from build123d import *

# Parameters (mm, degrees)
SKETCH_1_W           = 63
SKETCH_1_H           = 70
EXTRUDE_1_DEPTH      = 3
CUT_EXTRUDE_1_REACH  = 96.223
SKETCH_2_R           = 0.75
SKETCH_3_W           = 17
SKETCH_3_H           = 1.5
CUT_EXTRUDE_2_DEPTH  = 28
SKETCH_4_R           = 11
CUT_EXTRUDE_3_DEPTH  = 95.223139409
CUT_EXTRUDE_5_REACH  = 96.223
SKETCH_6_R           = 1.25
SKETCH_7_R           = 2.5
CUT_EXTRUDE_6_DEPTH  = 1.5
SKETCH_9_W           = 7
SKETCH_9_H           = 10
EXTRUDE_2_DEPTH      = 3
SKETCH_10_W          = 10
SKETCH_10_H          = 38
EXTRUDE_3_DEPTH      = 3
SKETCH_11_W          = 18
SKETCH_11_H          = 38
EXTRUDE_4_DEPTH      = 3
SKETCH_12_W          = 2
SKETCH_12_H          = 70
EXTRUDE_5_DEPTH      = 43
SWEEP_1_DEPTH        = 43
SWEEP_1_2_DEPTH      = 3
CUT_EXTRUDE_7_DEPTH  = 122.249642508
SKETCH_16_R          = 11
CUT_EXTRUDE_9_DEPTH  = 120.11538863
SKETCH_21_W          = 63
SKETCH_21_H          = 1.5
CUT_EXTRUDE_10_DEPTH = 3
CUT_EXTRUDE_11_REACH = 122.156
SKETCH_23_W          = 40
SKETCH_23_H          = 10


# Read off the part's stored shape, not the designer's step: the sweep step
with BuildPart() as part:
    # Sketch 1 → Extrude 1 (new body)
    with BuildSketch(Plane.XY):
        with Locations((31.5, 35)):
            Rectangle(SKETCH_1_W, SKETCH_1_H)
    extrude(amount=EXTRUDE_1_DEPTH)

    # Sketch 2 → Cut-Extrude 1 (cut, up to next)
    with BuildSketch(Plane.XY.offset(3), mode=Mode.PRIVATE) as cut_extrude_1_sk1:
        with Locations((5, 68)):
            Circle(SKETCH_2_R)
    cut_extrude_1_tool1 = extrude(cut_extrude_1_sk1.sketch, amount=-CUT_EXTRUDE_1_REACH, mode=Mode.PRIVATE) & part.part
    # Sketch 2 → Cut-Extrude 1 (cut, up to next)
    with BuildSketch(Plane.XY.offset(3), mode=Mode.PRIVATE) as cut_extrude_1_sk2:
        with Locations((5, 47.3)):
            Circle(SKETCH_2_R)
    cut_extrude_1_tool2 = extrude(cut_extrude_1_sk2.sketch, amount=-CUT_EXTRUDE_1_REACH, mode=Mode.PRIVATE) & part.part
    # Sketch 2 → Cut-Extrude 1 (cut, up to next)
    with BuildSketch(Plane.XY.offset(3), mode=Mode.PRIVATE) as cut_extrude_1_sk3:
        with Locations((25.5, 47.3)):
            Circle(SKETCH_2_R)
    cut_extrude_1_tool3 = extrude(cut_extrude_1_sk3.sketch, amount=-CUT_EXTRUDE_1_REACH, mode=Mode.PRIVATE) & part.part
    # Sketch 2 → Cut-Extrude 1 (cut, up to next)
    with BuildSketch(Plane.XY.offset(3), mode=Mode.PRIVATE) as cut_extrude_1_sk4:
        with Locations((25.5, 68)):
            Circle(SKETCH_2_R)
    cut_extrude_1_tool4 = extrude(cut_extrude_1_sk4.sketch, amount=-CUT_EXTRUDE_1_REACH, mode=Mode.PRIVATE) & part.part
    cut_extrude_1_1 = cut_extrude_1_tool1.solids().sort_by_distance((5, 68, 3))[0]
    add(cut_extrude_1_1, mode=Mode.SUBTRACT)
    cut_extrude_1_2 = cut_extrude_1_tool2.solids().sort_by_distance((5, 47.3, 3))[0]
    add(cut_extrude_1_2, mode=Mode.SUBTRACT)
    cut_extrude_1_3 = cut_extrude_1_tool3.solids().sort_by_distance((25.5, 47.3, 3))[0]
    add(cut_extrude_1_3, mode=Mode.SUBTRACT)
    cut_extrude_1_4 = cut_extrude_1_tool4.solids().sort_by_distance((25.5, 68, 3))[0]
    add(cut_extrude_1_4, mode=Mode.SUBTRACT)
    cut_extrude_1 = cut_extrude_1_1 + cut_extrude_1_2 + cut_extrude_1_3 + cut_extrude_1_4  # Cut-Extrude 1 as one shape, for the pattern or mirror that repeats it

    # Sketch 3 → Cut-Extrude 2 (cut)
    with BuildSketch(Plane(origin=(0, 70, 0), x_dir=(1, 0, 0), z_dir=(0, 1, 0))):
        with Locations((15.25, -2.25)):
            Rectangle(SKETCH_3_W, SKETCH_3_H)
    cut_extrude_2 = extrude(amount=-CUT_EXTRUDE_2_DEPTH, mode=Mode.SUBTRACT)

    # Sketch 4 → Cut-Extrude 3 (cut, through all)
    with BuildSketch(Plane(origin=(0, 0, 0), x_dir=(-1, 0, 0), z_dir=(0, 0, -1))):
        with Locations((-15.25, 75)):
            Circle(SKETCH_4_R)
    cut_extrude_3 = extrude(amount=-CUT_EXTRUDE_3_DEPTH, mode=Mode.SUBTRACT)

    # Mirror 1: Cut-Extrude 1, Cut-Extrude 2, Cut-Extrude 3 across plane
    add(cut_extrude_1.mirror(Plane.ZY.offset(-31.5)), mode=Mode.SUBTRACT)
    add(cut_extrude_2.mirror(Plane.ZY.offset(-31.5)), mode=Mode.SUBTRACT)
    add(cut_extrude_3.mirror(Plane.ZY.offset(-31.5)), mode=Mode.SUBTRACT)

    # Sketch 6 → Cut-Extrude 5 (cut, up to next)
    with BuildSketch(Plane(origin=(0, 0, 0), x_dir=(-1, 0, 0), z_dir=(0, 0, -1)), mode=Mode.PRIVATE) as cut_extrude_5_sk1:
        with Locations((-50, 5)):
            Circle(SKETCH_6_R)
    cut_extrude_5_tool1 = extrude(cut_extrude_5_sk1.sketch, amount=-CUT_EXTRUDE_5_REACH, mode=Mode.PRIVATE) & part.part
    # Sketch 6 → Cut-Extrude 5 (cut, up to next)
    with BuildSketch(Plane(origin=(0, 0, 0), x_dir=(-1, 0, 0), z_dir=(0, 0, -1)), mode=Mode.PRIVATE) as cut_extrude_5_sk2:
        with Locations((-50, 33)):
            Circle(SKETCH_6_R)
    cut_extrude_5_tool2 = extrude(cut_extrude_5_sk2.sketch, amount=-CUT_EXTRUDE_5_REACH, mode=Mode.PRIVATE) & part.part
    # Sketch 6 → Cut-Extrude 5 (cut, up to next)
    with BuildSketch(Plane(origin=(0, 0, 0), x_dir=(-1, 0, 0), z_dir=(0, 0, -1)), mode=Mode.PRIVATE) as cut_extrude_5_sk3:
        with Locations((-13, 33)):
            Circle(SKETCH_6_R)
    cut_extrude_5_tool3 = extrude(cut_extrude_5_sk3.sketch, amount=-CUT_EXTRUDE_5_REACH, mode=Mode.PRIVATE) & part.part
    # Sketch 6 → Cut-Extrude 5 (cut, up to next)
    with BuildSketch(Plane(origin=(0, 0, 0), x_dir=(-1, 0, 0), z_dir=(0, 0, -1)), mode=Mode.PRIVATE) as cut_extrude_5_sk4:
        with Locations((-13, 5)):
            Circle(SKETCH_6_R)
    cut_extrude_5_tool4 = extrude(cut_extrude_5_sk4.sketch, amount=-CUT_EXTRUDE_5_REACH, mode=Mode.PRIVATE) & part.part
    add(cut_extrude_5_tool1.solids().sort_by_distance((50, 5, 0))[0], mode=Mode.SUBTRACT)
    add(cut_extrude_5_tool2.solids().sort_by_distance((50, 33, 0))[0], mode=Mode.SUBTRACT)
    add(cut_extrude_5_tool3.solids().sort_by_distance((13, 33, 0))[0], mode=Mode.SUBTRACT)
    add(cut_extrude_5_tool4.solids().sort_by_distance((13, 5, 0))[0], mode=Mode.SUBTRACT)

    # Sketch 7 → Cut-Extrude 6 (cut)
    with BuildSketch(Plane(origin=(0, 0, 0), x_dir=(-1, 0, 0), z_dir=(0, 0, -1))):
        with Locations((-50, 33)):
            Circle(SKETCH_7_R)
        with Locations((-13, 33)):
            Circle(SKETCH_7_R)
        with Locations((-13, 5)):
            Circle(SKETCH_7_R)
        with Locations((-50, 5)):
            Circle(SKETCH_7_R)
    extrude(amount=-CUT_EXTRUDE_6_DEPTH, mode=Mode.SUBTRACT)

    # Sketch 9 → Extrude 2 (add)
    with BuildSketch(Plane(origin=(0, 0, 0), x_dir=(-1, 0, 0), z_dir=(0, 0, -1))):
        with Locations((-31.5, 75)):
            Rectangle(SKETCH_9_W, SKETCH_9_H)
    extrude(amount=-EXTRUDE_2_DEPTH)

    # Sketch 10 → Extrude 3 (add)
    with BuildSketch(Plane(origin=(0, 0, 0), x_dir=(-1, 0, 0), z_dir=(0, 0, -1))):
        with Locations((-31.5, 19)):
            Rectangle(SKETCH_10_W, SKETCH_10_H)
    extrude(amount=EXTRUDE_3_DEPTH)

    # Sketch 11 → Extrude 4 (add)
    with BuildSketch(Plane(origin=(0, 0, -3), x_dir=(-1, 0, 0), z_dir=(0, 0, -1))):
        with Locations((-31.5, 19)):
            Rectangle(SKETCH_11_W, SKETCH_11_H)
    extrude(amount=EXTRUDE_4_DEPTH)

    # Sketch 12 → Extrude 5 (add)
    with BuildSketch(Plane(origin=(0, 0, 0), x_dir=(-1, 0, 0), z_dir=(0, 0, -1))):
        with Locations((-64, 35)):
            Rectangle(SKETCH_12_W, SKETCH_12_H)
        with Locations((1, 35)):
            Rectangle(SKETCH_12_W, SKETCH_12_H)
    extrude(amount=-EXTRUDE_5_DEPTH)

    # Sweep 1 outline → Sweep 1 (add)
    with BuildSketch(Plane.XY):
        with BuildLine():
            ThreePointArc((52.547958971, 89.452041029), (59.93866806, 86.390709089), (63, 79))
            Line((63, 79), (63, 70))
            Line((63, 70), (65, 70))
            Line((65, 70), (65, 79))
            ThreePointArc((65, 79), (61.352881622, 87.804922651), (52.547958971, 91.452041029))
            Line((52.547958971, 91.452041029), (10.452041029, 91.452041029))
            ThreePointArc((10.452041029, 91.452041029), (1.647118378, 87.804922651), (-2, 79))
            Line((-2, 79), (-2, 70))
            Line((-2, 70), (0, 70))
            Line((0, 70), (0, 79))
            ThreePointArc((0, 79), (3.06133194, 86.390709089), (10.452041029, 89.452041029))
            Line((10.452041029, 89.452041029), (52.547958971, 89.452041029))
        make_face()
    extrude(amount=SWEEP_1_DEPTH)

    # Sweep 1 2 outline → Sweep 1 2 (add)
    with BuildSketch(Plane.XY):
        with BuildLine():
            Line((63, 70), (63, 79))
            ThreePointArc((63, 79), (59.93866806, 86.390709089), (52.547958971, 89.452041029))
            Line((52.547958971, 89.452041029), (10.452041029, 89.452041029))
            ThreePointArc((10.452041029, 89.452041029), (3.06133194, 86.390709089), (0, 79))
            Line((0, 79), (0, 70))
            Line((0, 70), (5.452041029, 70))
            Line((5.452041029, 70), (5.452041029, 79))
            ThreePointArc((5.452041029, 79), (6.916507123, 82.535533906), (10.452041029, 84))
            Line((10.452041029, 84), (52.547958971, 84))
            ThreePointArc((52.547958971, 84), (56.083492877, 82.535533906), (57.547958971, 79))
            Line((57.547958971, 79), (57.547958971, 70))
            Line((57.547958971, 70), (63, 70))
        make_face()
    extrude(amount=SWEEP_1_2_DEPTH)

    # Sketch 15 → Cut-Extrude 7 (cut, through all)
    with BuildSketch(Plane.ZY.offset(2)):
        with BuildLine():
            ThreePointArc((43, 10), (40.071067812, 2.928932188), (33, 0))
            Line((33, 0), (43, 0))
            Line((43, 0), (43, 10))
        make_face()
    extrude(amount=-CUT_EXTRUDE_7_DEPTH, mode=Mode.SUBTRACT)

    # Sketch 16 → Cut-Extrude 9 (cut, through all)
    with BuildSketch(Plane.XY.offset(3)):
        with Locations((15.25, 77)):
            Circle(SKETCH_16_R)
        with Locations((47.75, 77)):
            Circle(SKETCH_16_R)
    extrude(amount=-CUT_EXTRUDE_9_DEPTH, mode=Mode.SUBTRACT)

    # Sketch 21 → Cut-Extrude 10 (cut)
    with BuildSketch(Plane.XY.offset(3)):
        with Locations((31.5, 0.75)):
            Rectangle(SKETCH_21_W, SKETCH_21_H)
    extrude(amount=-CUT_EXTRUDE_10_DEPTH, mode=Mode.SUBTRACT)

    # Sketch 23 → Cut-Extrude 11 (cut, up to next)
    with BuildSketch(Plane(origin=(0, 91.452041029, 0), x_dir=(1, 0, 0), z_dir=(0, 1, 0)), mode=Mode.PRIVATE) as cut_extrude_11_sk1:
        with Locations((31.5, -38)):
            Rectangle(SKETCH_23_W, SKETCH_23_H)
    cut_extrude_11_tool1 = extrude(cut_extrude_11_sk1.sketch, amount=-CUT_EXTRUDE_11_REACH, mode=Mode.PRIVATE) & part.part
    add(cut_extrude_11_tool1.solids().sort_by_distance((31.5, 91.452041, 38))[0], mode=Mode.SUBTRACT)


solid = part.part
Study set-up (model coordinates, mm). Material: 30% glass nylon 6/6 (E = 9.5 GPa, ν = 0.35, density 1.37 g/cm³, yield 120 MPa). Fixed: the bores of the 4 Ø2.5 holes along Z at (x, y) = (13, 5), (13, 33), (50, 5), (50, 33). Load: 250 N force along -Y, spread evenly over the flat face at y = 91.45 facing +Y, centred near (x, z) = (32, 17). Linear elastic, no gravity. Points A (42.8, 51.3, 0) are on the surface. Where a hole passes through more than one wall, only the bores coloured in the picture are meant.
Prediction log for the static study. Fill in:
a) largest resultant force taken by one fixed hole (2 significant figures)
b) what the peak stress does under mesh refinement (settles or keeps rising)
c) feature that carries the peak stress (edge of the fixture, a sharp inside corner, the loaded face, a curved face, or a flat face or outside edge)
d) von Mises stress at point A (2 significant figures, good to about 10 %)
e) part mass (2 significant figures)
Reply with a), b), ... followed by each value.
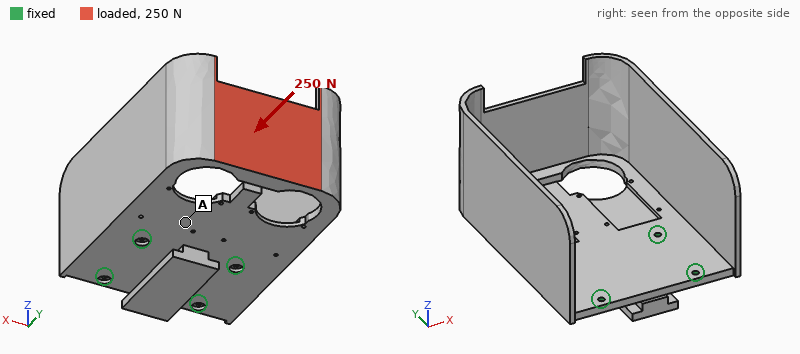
a) 130 N
b) keeps rising
c) edge of the fixture
d) 5.5 MPa
e) 48 g
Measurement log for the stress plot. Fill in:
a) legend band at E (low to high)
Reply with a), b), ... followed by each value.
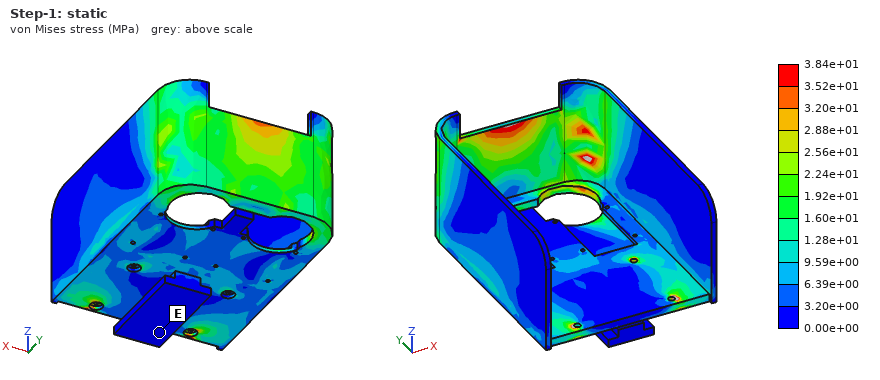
a) 0.00e+00 to 3.20e+00 MPa
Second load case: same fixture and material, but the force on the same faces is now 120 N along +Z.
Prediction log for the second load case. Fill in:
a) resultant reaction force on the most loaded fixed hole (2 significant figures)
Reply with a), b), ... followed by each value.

a) 220 N
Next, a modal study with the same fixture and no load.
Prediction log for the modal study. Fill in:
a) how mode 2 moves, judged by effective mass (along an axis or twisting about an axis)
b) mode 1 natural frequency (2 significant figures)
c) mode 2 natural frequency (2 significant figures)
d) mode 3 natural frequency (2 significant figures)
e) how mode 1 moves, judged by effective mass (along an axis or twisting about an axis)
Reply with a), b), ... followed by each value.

a) along Z
b) 340 Hz
c) 400 Hz
d) 490 Hz
e) along X
